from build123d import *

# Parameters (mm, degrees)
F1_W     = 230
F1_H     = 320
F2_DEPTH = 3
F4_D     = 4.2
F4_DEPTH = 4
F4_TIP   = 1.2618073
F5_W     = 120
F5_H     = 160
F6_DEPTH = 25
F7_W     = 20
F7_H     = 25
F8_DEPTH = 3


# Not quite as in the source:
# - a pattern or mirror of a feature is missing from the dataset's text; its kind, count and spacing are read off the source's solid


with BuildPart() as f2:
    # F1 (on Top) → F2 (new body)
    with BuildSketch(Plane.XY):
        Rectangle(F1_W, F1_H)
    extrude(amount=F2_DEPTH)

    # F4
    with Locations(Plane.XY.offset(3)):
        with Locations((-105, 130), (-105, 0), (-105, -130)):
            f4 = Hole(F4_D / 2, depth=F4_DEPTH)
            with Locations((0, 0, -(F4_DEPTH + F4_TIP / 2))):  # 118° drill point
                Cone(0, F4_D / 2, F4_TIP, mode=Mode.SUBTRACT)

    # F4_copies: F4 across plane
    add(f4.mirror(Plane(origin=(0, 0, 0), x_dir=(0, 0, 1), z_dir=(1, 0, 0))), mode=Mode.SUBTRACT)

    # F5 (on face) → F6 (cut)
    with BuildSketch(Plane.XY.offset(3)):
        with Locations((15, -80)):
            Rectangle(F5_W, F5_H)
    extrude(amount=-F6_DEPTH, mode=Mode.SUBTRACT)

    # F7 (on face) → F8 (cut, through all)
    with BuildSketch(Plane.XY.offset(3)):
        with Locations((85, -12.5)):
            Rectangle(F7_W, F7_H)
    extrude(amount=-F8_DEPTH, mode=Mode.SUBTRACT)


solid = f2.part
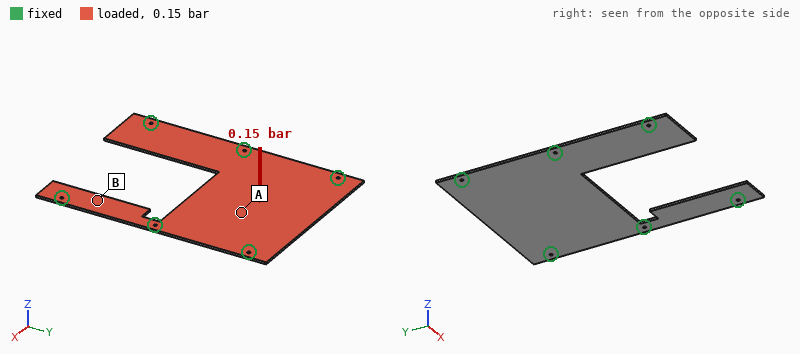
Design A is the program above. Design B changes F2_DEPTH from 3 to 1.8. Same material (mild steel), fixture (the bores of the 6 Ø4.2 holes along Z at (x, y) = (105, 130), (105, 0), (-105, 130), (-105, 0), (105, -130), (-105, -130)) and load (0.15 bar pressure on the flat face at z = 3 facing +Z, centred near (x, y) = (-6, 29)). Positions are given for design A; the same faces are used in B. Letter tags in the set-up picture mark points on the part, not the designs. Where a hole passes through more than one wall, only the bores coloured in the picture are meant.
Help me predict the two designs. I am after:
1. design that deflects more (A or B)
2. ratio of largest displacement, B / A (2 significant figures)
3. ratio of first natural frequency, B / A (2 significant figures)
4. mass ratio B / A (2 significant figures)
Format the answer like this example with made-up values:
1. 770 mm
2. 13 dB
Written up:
1. B
2. 4.5
3. 0.61
4. 0.60
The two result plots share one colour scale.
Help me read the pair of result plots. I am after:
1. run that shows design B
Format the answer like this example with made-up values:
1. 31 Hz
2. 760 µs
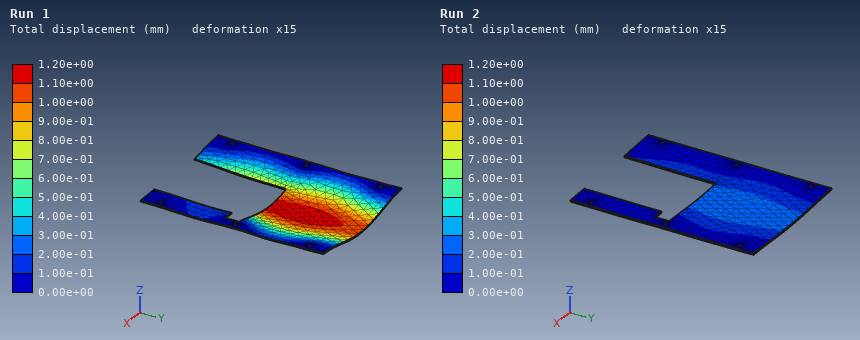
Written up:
1. Run 1
